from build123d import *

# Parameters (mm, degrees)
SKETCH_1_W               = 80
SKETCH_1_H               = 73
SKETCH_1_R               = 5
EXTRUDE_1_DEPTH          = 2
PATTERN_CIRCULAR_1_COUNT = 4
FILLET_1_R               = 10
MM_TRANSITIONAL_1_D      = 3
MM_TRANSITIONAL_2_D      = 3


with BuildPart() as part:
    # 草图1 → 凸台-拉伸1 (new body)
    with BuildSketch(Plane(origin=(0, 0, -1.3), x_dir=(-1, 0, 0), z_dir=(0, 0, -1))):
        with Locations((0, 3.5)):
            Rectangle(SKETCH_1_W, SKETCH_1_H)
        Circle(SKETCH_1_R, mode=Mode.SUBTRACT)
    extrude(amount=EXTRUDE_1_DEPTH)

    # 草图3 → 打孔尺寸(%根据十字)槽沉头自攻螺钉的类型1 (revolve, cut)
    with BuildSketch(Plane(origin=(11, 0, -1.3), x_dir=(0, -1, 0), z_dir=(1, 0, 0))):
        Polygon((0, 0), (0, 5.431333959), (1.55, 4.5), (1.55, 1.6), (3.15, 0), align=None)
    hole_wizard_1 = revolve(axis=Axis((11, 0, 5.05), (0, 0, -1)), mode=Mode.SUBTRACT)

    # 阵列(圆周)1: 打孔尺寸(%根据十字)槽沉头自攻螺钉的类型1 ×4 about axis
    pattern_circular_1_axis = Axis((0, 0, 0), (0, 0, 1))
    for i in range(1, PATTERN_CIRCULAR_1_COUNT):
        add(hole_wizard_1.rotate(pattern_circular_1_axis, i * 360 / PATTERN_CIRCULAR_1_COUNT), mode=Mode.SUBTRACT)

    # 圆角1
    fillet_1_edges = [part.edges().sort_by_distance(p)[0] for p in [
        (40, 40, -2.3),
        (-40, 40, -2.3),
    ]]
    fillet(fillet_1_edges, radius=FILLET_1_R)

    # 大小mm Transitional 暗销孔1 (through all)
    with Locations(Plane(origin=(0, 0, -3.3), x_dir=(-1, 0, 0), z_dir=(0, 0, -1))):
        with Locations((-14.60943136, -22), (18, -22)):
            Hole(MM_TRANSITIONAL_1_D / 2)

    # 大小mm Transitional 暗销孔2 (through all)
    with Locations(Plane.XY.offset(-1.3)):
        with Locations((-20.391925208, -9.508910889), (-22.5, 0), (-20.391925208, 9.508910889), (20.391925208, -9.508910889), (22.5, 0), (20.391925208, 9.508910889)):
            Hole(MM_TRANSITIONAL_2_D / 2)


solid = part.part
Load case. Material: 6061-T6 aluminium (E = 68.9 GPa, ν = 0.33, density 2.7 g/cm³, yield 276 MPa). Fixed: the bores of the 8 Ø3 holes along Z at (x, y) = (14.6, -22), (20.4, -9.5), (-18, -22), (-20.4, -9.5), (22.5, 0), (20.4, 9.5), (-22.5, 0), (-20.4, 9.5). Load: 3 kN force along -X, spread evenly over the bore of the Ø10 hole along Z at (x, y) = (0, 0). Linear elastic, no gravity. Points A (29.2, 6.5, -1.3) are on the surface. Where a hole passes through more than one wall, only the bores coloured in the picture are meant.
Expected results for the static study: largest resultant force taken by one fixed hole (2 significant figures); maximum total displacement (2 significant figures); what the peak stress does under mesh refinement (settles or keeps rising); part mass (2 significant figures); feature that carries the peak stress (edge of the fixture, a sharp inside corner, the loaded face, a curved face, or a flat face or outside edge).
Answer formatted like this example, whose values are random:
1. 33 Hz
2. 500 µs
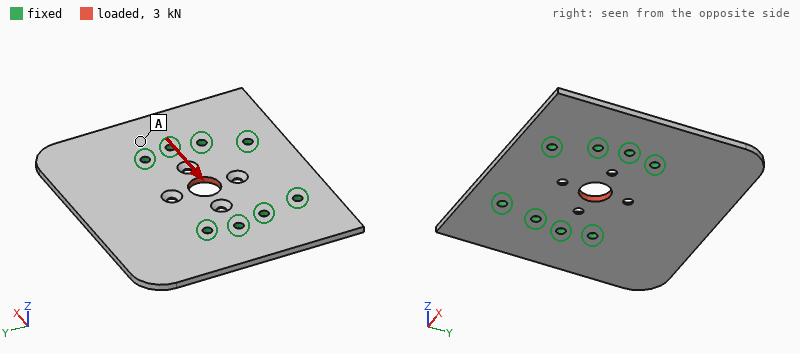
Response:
1. 590 N
2. 12 µm
3. keeps rising
4. 30 g
5. a sharp inside corner
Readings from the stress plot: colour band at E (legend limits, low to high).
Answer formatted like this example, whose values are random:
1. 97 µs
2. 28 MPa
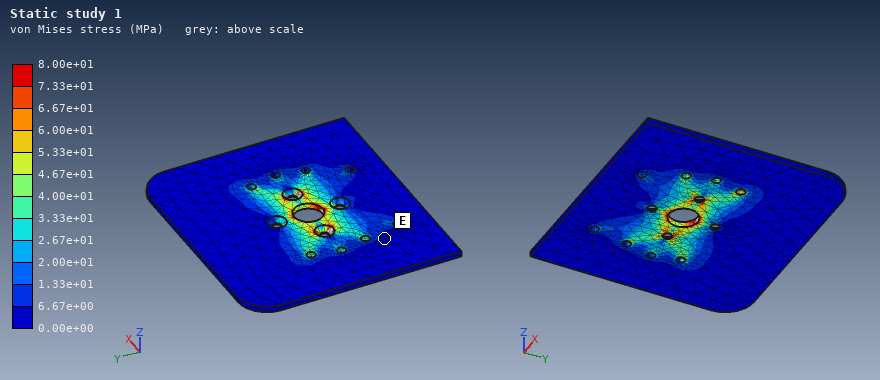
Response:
1. 0.00e+00 to 6.67e+00 MPa
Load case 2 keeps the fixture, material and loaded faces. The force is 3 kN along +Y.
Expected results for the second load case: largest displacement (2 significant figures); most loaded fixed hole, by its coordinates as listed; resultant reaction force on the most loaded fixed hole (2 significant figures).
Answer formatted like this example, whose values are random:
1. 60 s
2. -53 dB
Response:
1. 16 µm
2. (14.6, -22)
3. 630 N
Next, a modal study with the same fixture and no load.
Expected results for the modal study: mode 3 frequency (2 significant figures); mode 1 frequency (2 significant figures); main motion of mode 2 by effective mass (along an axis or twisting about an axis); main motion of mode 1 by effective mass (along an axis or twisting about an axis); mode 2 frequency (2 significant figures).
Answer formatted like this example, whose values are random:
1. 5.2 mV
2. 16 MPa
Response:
1. 3000 Hz
2. 1600 Hz
3. twisting about Y
4. along Z
5. 2100 Hz
